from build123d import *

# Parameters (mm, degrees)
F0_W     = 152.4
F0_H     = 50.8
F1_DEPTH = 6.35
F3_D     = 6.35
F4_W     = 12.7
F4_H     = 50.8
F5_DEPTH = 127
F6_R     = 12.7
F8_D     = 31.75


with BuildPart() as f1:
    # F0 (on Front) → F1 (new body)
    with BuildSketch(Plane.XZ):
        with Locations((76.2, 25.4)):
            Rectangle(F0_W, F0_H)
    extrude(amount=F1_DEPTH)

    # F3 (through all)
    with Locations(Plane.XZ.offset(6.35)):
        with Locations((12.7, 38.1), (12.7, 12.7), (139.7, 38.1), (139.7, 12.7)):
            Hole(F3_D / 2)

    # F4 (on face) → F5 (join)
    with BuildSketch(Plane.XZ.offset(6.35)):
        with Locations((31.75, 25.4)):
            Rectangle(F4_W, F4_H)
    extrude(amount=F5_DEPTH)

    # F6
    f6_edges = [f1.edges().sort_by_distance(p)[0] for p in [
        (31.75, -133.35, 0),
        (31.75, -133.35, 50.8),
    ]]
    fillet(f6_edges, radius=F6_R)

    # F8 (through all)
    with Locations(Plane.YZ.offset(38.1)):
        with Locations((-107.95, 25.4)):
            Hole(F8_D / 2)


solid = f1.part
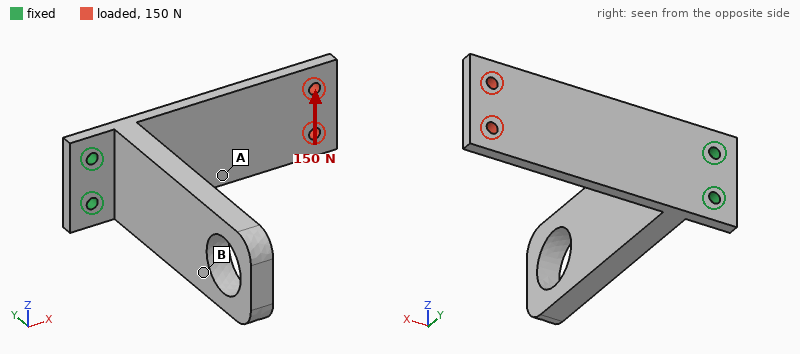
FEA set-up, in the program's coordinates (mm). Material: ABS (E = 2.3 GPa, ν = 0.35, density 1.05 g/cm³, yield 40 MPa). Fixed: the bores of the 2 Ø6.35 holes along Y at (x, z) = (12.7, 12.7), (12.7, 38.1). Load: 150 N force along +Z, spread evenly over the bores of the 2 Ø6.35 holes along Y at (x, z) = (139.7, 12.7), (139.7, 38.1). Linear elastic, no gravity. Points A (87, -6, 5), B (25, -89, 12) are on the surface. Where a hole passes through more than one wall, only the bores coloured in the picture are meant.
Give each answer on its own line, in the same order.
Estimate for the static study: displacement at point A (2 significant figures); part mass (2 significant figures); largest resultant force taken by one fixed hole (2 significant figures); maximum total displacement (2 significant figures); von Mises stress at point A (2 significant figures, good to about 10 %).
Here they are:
0.39 mm
130 g
650 N
0.94 mm
2.3 MPa
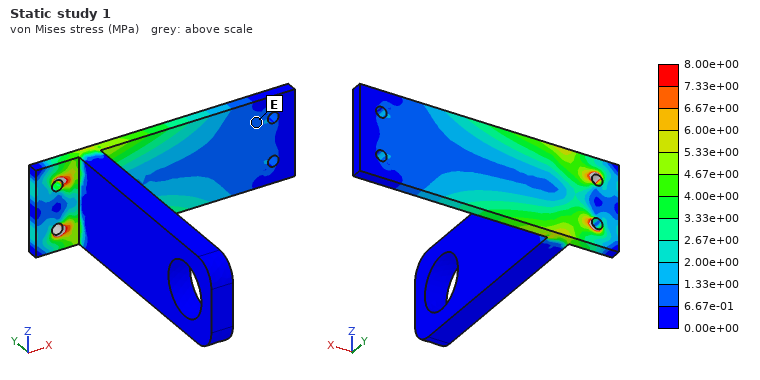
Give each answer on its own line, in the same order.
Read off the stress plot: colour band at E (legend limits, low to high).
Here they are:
6.67e-01 to 1.33e+00 MPa
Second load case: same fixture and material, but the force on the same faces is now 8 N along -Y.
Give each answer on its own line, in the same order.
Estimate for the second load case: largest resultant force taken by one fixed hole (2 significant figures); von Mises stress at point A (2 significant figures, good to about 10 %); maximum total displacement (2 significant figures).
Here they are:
4.1 N
1.2 MPa
2.1 mm
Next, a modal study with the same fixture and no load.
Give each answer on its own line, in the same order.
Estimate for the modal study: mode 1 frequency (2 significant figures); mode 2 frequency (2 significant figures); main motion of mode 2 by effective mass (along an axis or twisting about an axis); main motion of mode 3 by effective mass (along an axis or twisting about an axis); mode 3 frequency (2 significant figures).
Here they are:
73 Hz
140 Hz
along X
along Z
240 Hz
